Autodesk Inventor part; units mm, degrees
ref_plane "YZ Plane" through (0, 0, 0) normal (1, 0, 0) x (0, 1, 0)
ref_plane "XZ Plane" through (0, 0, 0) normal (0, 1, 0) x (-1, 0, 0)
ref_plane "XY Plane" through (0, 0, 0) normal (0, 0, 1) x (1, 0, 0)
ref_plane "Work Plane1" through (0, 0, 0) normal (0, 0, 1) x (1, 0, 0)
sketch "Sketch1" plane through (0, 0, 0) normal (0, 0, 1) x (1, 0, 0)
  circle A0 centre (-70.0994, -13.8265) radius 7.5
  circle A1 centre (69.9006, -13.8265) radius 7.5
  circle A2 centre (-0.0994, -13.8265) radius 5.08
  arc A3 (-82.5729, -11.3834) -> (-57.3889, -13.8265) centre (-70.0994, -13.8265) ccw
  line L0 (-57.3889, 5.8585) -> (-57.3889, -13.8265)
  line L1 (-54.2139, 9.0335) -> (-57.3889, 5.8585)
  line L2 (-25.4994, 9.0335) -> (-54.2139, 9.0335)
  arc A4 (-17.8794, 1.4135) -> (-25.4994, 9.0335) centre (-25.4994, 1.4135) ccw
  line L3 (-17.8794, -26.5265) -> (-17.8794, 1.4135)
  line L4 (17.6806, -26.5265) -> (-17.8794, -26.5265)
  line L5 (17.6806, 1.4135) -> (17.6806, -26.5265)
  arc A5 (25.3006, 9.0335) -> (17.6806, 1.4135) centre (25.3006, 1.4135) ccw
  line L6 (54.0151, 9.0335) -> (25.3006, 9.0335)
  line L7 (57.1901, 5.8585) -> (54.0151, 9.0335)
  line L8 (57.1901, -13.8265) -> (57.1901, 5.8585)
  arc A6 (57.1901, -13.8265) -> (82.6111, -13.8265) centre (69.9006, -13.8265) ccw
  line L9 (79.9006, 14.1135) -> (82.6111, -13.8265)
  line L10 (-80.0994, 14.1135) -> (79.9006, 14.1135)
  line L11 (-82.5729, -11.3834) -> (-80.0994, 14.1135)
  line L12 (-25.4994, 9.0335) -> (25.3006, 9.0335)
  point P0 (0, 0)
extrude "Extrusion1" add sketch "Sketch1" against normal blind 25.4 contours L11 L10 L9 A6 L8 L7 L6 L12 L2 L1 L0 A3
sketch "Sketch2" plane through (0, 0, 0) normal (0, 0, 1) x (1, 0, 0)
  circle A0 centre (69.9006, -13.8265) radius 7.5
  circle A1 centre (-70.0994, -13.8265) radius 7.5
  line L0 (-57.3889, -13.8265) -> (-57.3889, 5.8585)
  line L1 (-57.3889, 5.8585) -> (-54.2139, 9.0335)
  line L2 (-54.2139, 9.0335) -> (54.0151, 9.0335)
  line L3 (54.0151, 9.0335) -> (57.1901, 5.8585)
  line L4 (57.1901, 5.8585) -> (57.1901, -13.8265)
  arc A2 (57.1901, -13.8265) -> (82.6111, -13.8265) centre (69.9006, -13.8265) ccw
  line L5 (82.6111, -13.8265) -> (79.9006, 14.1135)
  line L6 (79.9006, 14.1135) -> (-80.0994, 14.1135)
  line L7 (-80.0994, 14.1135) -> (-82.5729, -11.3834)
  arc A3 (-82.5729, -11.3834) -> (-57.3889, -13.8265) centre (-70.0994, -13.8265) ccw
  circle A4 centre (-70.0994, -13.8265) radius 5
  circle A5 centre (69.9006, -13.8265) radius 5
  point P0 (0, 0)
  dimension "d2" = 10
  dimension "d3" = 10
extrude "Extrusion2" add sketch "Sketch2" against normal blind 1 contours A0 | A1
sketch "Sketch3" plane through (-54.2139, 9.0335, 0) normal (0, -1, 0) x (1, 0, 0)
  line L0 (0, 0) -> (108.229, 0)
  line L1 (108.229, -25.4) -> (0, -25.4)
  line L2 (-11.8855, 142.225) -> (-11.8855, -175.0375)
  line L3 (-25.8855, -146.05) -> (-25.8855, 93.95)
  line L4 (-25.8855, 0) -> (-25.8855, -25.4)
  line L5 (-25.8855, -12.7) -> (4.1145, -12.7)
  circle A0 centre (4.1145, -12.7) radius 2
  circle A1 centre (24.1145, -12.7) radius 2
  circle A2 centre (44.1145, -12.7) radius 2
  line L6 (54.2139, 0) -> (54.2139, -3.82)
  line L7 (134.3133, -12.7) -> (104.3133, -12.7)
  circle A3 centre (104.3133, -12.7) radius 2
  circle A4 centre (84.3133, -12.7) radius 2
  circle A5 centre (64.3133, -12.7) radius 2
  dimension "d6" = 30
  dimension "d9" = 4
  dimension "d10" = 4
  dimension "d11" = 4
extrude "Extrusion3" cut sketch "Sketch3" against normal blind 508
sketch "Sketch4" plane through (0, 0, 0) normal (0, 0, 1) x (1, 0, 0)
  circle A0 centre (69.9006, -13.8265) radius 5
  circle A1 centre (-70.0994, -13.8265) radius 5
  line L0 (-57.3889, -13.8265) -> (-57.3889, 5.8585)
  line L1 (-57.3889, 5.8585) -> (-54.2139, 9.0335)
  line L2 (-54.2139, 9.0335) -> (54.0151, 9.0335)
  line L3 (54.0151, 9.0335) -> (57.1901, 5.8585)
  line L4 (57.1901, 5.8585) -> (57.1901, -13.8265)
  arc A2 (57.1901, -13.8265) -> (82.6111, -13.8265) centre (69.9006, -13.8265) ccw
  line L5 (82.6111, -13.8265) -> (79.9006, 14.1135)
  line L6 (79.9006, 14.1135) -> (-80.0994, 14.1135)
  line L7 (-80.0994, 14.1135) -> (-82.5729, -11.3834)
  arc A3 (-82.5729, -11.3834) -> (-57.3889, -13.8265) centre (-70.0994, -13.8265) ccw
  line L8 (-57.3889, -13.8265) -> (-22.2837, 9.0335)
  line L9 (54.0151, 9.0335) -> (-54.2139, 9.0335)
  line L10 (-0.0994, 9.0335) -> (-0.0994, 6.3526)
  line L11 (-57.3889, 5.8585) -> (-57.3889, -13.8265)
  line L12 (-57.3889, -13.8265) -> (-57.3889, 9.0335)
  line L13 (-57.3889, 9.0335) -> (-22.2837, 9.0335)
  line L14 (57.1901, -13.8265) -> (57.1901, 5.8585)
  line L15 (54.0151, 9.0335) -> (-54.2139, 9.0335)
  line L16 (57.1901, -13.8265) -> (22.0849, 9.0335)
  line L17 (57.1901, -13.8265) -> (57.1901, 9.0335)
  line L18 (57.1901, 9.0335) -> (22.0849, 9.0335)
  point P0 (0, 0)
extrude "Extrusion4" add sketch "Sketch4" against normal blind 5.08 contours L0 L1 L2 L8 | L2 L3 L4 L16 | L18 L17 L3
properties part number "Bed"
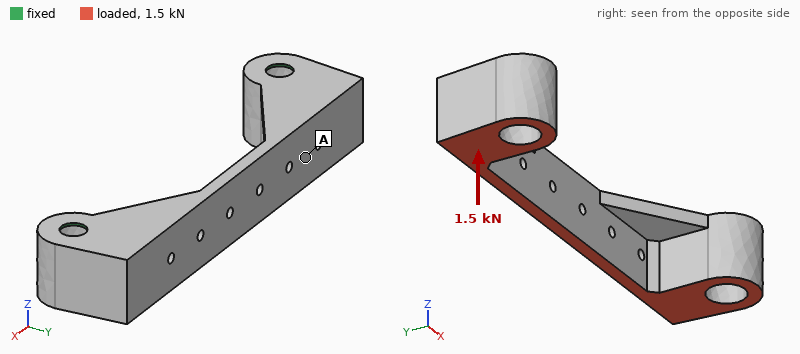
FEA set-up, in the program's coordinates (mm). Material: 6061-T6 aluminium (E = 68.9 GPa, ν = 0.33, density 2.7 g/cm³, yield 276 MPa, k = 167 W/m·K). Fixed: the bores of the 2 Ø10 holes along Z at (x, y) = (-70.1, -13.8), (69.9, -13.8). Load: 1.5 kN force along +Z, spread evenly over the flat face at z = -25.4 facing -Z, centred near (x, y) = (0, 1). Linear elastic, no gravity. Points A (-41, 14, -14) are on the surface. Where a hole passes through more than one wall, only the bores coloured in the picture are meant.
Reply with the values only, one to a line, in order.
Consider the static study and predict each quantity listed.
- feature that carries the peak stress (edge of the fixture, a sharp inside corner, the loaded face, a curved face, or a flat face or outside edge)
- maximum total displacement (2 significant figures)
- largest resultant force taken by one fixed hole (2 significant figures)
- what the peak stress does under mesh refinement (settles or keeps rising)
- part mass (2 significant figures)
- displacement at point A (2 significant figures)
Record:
edge of the fixture
0.20 mm
760 N
keeps rising
150 g
0.16 mm
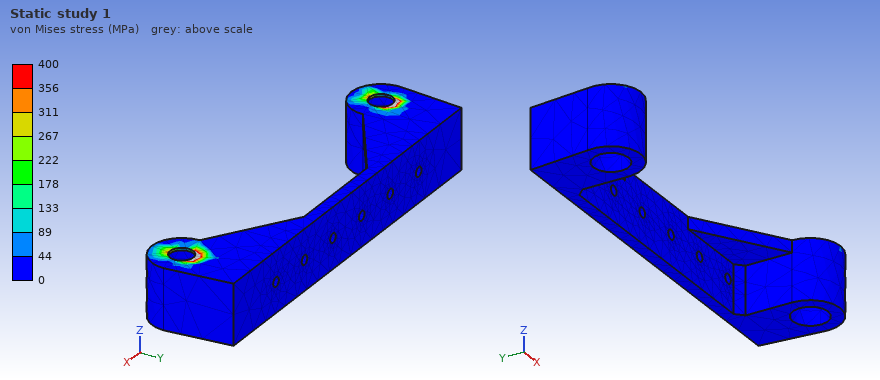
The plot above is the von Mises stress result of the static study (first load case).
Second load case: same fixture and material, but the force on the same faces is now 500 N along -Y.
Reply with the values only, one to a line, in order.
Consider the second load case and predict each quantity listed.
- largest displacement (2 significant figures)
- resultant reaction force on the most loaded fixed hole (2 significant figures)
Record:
0.12 mm
260 N
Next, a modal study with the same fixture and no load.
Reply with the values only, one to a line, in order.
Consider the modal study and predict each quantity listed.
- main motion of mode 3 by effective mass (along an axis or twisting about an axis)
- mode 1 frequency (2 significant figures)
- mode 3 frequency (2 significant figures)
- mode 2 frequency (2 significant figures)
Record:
along X
1200 Hz
3200 Hz
1700 Hz
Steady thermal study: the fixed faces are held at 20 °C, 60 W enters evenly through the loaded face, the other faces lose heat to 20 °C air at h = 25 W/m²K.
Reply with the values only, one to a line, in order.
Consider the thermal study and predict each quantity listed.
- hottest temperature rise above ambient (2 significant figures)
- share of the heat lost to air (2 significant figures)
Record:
28 K
14 %
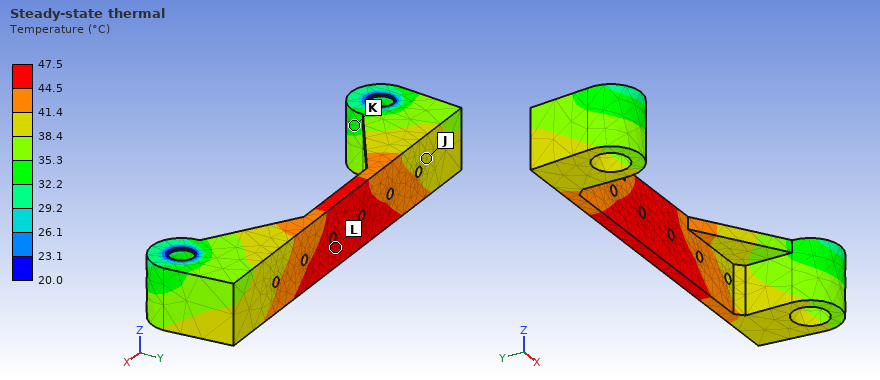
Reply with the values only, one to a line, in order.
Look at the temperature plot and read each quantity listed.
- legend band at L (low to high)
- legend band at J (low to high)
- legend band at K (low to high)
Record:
44.5 to 47.5 °C
38.4 to 41.4 °C
32.2 to 35.3 °C
